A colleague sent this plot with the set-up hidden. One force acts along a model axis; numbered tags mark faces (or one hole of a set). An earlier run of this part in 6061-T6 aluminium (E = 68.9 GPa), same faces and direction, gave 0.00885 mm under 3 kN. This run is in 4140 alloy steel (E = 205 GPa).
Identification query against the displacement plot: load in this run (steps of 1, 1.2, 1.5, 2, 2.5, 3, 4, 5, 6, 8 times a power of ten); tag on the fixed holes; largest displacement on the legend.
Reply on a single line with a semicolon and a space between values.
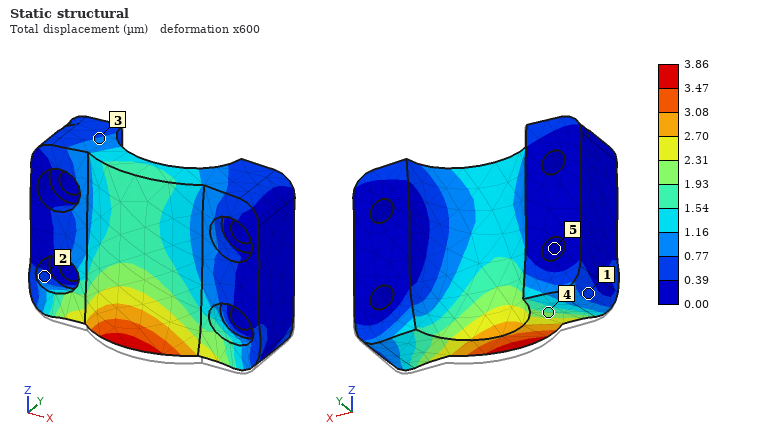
4 kN; 5; 3.86 µm
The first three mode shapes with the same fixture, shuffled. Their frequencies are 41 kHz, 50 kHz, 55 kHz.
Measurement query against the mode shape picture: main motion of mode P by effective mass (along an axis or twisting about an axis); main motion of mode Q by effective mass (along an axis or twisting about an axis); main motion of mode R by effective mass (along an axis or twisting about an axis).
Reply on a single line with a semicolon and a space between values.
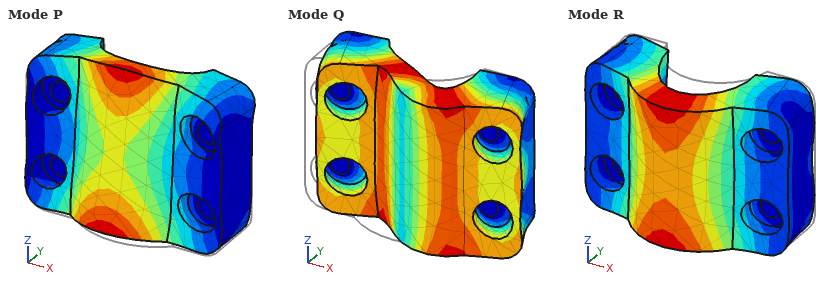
along Z; along X; along Y
